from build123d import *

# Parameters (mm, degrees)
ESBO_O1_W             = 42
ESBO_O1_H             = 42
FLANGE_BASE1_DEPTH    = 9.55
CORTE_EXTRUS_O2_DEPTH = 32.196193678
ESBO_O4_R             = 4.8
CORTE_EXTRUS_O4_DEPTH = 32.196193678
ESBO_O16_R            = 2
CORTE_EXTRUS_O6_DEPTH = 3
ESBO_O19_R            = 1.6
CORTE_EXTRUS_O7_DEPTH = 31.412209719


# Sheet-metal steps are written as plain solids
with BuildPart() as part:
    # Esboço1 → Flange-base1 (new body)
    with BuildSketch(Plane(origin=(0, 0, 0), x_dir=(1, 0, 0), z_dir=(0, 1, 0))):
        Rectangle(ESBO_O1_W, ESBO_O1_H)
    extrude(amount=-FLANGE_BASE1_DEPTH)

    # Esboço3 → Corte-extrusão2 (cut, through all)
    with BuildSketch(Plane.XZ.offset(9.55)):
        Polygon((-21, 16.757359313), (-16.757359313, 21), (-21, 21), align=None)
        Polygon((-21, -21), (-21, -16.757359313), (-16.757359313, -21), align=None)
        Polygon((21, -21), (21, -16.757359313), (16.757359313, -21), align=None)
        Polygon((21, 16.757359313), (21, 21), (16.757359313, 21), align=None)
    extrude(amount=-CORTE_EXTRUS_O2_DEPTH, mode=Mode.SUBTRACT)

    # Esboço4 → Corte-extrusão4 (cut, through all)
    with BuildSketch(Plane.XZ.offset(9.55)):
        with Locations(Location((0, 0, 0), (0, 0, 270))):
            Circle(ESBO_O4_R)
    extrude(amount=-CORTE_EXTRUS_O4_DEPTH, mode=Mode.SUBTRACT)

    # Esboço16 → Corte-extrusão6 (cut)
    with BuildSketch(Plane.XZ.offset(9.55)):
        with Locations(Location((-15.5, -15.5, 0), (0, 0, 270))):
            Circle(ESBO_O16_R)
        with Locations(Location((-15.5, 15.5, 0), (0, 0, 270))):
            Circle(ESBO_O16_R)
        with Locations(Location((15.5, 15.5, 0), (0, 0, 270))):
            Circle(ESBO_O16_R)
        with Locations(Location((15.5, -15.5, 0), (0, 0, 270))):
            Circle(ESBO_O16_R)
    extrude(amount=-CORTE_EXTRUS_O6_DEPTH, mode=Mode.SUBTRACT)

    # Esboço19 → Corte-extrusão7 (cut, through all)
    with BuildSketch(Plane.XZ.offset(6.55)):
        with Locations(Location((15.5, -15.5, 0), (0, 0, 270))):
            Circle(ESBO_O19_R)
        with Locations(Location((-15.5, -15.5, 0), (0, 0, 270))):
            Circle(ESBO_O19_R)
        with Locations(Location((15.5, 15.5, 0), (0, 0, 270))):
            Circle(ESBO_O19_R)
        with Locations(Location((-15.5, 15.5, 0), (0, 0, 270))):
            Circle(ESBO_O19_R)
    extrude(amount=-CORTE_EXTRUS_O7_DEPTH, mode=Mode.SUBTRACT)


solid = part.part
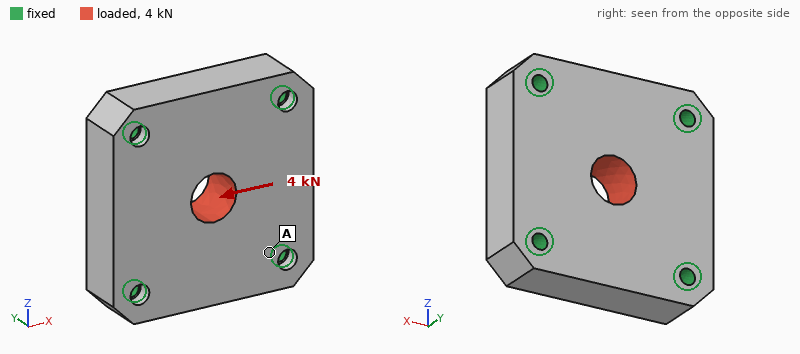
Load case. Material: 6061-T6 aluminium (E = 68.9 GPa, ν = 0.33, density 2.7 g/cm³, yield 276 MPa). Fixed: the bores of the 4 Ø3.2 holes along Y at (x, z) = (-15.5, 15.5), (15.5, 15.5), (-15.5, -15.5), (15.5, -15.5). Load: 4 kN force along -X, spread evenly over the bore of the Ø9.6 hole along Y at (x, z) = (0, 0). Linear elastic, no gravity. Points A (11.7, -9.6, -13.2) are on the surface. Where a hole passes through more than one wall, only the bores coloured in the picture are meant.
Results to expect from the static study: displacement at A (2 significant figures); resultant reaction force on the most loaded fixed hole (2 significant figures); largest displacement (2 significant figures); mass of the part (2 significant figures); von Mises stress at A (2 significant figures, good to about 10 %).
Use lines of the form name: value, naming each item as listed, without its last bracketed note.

displacement at A: 1.4 µm
resultant reaction force on the most loaded fixed hole: 1.1 kN
largest displacement: 4.5 µm
mass of the part: 42 g
von Mises stress at A: 5.6 MPa
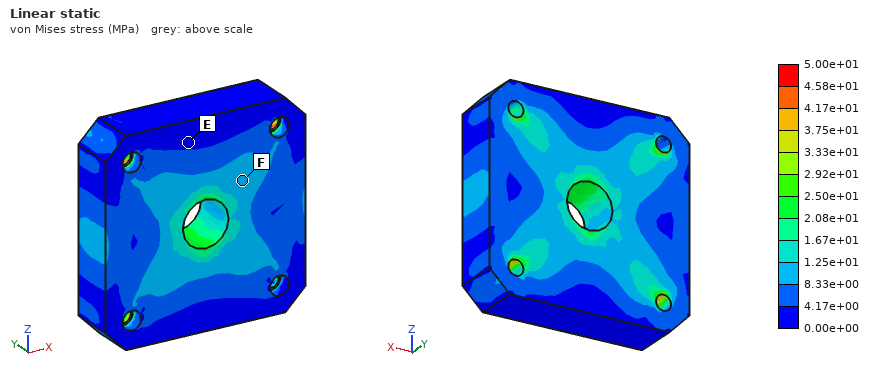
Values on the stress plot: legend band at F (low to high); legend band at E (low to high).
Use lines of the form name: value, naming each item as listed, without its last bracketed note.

legend band at F: 8.33e+00 to 1.25e+01 MPa
legend band at E: 0.00e+00 to 4.17e+00 MPa
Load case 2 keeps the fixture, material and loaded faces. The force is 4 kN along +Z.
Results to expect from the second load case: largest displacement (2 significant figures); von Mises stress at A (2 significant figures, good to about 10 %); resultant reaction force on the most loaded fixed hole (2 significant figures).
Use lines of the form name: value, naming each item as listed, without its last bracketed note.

largest displacement: 4.5 µm
von Mises stress at A: 7.8 MPa
resultant reaction force on the most loaded fixed hole: 1.1 kN
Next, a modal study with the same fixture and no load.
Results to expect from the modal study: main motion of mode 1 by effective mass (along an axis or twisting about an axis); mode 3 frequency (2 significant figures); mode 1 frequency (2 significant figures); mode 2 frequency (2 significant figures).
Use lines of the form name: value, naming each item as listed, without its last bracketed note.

main motion of mode 1 by effective mass: along Y
mode 3 frequency: 32 kHz
mode 1 frequency: 22 kHz
mode 2 frequency: 32 kHz
